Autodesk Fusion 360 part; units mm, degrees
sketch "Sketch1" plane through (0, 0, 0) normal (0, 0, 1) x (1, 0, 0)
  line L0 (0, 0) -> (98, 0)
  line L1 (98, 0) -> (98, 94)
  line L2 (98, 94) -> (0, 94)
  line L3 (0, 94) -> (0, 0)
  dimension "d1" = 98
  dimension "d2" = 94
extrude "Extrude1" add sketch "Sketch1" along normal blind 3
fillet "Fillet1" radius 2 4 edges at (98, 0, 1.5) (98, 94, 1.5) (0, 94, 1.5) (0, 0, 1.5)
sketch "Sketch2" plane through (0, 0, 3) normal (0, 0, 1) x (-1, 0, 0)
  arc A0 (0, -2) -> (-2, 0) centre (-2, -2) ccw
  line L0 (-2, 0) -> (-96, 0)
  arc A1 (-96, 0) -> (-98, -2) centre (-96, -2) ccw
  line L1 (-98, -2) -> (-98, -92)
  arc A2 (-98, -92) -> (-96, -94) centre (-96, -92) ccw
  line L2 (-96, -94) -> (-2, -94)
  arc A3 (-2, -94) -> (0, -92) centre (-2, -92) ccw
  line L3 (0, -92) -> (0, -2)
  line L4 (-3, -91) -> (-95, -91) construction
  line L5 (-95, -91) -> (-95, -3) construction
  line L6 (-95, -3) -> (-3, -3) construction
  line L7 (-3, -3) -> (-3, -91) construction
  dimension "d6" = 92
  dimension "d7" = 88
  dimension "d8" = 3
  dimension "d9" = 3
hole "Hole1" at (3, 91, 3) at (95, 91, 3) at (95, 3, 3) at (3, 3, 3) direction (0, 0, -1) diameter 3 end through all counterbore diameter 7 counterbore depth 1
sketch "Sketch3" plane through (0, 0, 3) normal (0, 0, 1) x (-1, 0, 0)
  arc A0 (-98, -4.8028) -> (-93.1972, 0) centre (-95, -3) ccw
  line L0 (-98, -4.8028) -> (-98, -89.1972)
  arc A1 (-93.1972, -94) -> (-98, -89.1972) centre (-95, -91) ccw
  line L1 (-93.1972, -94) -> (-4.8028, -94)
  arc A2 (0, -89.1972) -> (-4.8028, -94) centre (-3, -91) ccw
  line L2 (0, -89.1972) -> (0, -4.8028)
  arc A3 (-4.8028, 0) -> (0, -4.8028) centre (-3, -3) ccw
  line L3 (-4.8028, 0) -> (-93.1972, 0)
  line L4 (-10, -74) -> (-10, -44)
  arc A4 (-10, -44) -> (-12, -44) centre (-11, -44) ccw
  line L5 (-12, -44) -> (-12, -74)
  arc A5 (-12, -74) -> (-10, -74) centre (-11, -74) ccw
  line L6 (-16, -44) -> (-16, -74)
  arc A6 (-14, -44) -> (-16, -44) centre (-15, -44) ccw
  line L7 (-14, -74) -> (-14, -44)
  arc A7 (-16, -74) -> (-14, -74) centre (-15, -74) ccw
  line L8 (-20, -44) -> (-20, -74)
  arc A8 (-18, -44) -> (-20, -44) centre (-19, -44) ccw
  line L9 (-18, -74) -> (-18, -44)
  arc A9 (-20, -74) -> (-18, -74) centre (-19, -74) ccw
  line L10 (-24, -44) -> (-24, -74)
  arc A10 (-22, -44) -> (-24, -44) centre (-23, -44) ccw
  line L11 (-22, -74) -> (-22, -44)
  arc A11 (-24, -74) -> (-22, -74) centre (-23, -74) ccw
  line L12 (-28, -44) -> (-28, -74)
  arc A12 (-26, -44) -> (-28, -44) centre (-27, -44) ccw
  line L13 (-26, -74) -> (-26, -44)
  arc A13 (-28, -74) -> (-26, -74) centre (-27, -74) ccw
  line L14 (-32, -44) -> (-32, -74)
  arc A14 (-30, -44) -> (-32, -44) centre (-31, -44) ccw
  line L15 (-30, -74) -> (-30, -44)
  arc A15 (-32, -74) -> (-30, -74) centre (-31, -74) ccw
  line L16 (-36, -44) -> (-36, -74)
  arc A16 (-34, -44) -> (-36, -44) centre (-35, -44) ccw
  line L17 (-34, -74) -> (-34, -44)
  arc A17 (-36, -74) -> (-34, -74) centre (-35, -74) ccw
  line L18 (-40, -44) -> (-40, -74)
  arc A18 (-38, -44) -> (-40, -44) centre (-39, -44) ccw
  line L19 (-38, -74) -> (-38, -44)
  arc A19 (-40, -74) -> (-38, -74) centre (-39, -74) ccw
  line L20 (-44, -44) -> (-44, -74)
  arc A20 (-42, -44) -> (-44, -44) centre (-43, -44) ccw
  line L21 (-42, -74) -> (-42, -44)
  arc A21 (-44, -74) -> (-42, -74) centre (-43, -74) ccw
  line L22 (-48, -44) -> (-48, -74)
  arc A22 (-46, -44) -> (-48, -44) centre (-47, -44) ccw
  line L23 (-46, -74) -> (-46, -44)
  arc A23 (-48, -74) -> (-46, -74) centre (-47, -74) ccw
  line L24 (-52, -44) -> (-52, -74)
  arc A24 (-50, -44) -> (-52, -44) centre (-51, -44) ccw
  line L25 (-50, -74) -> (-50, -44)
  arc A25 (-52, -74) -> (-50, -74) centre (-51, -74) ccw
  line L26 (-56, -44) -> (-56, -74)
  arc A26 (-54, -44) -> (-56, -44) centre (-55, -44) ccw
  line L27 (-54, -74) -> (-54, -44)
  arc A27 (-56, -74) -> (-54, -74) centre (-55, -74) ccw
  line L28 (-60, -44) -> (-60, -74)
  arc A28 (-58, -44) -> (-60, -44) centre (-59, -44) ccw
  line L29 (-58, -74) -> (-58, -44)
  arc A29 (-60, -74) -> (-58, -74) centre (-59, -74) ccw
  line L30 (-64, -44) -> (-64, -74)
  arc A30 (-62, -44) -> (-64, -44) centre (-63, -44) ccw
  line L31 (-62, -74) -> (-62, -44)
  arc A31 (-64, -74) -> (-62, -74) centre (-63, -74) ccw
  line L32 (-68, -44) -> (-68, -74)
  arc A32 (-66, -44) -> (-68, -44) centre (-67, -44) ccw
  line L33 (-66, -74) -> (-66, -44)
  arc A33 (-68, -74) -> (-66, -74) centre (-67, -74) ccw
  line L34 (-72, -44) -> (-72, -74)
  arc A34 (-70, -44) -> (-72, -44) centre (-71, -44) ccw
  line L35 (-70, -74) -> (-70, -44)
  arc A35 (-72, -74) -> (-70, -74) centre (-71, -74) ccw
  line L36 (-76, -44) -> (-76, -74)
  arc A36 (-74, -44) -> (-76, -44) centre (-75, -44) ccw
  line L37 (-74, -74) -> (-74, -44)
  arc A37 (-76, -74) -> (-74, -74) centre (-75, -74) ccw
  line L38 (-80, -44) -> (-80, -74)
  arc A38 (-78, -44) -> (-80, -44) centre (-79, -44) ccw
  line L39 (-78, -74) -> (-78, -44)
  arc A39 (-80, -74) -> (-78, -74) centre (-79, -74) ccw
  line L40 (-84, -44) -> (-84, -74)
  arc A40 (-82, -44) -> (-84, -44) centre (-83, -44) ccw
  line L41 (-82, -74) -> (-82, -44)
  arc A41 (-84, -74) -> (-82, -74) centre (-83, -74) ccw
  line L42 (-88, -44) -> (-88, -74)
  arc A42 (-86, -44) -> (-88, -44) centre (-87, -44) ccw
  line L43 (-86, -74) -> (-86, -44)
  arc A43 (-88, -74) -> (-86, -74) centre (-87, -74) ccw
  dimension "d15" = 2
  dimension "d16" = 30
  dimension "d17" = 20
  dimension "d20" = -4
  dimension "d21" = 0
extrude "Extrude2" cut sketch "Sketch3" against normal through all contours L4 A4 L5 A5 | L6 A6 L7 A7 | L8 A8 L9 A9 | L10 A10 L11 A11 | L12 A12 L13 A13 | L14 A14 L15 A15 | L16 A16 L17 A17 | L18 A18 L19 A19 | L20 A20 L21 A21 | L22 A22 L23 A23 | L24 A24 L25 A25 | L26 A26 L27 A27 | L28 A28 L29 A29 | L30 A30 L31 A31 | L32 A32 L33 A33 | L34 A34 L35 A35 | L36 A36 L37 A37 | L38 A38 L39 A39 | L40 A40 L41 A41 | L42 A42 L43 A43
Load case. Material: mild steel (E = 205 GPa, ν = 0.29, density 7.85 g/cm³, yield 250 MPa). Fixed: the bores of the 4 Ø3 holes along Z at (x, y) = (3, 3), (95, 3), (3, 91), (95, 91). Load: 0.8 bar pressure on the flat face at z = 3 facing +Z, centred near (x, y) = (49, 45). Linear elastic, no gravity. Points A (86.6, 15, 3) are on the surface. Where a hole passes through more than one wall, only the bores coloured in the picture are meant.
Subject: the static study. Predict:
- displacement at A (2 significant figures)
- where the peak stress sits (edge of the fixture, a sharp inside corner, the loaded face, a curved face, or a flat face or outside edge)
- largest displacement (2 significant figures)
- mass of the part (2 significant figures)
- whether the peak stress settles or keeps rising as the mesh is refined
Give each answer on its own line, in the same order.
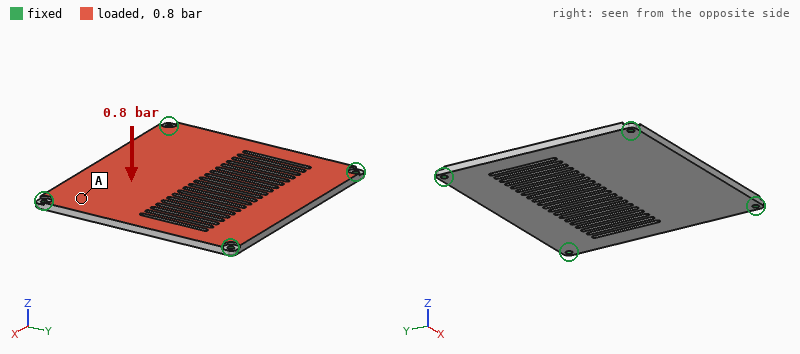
0.038 mm
edge of the fixture
0.15 mm
190 g
keeps rising
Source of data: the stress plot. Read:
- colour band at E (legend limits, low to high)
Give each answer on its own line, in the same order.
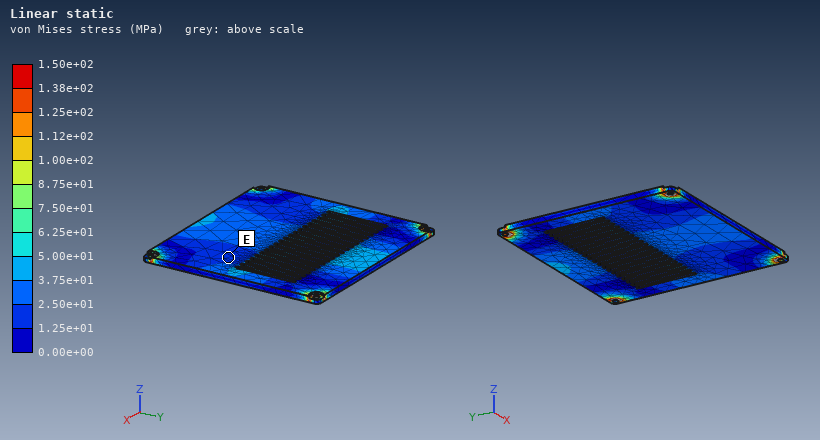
1.25e+01 to 2.50e+01 MPa
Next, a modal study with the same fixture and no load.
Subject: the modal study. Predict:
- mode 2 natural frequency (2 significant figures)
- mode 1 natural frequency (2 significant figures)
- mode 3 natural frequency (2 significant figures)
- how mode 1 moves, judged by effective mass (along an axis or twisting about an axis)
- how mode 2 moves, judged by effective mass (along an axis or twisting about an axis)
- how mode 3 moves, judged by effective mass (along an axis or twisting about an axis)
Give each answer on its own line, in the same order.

1700 Hz
950 Hz
1900 Hz
along Z
twisting about X
twisting about Y
